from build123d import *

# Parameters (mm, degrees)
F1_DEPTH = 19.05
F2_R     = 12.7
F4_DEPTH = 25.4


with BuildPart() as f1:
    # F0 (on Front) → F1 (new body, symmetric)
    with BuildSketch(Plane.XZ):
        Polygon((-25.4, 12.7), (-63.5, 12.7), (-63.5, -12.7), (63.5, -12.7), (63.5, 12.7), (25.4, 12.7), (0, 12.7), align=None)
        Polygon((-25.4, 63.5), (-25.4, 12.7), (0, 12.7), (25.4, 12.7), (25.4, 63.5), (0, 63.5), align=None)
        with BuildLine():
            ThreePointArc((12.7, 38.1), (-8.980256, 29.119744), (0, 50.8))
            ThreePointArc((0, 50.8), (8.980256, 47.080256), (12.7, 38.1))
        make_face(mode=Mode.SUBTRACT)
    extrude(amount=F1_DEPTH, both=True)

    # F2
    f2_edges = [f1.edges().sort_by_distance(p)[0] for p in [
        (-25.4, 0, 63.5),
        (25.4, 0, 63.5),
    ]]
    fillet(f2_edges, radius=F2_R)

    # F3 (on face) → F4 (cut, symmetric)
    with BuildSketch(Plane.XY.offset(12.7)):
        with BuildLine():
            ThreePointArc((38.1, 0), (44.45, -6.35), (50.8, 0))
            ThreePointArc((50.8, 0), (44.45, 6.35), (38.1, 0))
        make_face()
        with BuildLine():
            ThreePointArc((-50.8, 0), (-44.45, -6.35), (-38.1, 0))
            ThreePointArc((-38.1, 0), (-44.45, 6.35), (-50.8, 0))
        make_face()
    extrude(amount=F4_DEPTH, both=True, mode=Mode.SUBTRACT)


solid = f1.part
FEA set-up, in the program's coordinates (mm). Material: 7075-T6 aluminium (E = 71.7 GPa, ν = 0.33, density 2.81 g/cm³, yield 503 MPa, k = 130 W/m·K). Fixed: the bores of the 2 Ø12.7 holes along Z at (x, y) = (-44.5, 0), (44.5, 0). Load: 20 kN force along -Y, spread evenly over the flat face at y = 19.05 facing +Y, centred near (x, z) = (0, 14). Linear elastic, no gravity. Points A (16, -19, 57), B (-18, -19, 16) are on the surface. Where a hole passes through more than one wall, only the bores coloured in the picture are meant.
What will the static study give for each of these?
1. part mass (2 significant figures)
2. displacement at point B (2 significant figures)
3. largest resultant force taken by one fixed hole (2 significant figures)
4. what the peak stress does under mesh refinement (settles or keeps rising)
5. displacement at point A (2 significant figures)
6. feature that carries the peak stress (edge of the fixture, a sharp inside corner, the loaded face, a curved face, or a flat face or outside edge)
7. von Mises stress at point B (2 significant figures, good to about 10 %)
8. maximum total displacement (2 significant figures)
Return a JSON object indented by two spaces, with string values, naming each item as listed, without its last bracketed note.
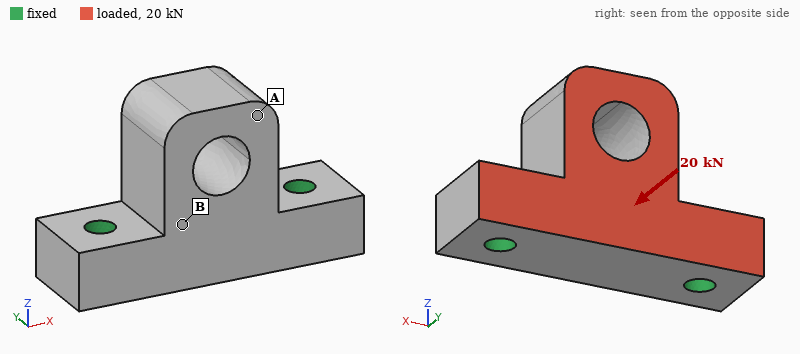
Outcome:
{
  "part mass": "540 g",
  "displacement at point B": "0.035 mm",
  "largest resultant force taken by one fixed hole": "10 kN",
  "what the peak stress does under mesh refinement": "keeps rising",
  "displacement at point A": "0.090 mm",
  "feature that carries the peak stress": "edge of the fixture",
  "von Mises stress at point B": "18 MPa",
  "maximum total displacement": "0.10 mm"
}
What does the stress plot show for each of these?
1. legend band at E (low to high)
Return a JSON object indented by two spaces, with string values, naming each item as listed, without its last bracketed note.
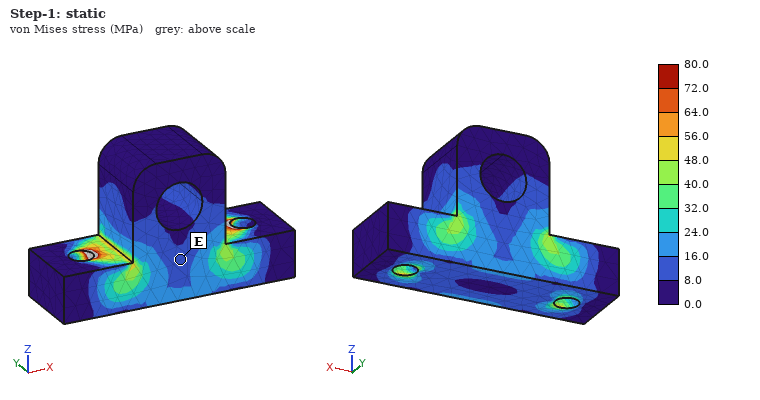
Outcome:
{
  "legend band at E": "8.0 to 16.0 MPa"
}
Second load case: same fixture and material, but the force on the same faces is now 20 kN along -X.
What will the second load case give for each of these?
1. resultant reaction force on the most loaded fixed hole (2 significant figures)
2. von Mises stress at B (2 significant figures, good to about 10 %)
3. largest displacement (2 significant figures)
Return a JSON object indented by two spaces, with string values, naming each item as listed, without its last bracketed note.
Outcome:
{
  "resultant reaction force on the most loaded fixed hole": "11 kN",
  "von Mises stress at B": "7.3 MPa",
  "largest displacement": "45 µm"
}
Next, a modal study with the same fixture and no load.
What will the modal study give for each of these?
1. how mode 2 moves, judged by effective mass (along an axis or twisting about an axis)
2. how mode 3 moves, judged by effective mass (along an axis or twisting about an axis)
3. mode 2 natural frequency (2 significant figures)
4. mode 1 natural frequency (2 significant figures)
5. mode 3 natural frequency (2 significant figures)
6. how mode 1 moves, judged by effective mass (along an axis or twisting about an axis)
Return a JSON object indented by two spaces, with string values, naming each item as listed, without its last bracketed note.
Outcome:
{
  "how mode 2 moves, judged by effective mass": "along X",
  "how mode 3 moves, judged by effective mass": "along Z",
  "mode 2 natural frequency": "6300 Hz",
  "mode 1 natural frequency": "3600 Hz",
  "mode 3 natural frequency": "9000 Hz",
  "how mode 1 moves, judged by effective mass": "along Y"
}
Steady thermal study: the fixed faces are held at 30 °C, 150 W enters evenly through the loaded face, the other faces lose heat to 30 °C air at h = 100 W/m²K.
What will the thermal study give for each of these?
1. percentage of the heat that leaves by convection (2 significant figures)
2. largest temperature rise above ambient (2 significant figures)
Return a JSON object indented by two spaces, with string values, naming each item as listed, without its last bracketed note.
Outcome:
{
  "percentage of the heat that leaves by convection": "13 %",
  "largest temperature rise above ambient": "19 K"
}
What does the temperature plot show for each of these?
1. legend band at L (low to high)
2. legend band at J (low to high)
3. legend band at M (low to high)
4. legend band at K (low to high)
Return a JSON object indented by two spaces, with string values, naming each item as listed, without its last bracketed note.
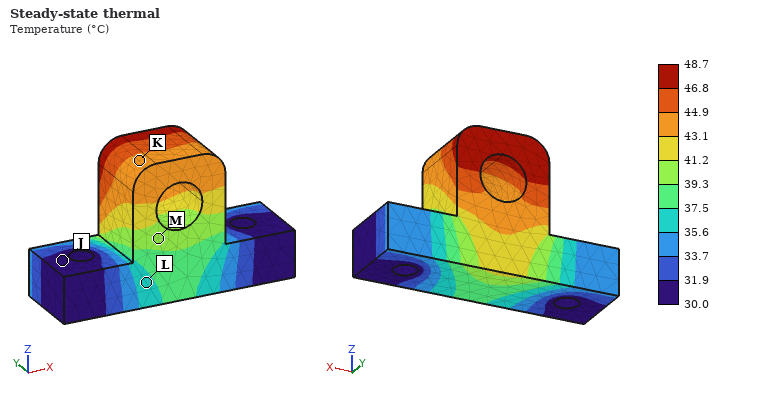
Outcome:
{
  "legend band at L": "35.6 to 37.5 °C",
  "legend band at J": "30.0 to 31.9 °C",
  "legend band at M": "39.3 to 41.2 °C",
  "legend band at K": "43.1 to 44.9 °C"
}
